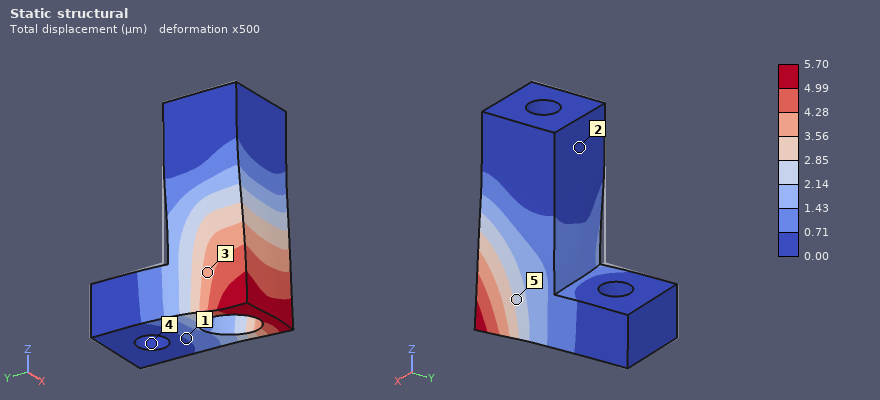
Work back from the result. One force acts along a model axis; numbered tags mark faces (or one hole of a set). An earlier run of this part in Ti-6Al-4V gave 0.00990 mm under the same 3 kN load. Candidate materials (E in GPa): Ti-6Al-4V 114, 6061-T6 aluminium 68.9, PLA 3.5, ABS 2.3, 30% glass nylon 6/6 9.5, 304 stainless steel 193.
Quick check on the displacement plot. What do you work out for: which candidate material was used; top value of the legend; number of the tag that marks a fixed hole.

304 stainless steel
5.70 µm
4
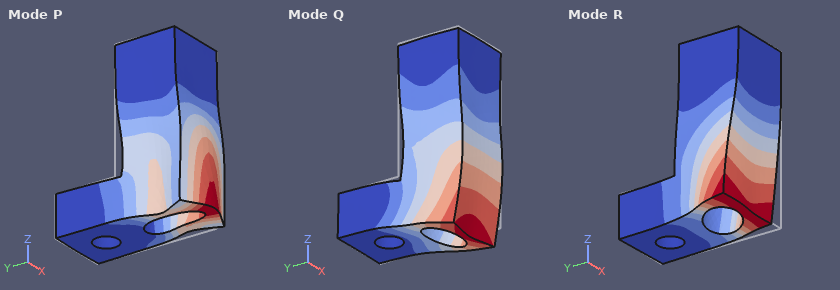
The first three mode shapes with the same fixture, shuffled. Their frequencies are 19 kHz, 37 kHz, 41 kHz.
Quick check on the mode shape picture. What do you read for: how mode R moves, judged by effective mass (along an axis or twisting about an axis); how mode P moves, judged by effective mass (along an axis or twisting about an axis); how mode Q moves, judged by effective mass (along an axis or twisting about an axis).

along X
along Y
along Z
